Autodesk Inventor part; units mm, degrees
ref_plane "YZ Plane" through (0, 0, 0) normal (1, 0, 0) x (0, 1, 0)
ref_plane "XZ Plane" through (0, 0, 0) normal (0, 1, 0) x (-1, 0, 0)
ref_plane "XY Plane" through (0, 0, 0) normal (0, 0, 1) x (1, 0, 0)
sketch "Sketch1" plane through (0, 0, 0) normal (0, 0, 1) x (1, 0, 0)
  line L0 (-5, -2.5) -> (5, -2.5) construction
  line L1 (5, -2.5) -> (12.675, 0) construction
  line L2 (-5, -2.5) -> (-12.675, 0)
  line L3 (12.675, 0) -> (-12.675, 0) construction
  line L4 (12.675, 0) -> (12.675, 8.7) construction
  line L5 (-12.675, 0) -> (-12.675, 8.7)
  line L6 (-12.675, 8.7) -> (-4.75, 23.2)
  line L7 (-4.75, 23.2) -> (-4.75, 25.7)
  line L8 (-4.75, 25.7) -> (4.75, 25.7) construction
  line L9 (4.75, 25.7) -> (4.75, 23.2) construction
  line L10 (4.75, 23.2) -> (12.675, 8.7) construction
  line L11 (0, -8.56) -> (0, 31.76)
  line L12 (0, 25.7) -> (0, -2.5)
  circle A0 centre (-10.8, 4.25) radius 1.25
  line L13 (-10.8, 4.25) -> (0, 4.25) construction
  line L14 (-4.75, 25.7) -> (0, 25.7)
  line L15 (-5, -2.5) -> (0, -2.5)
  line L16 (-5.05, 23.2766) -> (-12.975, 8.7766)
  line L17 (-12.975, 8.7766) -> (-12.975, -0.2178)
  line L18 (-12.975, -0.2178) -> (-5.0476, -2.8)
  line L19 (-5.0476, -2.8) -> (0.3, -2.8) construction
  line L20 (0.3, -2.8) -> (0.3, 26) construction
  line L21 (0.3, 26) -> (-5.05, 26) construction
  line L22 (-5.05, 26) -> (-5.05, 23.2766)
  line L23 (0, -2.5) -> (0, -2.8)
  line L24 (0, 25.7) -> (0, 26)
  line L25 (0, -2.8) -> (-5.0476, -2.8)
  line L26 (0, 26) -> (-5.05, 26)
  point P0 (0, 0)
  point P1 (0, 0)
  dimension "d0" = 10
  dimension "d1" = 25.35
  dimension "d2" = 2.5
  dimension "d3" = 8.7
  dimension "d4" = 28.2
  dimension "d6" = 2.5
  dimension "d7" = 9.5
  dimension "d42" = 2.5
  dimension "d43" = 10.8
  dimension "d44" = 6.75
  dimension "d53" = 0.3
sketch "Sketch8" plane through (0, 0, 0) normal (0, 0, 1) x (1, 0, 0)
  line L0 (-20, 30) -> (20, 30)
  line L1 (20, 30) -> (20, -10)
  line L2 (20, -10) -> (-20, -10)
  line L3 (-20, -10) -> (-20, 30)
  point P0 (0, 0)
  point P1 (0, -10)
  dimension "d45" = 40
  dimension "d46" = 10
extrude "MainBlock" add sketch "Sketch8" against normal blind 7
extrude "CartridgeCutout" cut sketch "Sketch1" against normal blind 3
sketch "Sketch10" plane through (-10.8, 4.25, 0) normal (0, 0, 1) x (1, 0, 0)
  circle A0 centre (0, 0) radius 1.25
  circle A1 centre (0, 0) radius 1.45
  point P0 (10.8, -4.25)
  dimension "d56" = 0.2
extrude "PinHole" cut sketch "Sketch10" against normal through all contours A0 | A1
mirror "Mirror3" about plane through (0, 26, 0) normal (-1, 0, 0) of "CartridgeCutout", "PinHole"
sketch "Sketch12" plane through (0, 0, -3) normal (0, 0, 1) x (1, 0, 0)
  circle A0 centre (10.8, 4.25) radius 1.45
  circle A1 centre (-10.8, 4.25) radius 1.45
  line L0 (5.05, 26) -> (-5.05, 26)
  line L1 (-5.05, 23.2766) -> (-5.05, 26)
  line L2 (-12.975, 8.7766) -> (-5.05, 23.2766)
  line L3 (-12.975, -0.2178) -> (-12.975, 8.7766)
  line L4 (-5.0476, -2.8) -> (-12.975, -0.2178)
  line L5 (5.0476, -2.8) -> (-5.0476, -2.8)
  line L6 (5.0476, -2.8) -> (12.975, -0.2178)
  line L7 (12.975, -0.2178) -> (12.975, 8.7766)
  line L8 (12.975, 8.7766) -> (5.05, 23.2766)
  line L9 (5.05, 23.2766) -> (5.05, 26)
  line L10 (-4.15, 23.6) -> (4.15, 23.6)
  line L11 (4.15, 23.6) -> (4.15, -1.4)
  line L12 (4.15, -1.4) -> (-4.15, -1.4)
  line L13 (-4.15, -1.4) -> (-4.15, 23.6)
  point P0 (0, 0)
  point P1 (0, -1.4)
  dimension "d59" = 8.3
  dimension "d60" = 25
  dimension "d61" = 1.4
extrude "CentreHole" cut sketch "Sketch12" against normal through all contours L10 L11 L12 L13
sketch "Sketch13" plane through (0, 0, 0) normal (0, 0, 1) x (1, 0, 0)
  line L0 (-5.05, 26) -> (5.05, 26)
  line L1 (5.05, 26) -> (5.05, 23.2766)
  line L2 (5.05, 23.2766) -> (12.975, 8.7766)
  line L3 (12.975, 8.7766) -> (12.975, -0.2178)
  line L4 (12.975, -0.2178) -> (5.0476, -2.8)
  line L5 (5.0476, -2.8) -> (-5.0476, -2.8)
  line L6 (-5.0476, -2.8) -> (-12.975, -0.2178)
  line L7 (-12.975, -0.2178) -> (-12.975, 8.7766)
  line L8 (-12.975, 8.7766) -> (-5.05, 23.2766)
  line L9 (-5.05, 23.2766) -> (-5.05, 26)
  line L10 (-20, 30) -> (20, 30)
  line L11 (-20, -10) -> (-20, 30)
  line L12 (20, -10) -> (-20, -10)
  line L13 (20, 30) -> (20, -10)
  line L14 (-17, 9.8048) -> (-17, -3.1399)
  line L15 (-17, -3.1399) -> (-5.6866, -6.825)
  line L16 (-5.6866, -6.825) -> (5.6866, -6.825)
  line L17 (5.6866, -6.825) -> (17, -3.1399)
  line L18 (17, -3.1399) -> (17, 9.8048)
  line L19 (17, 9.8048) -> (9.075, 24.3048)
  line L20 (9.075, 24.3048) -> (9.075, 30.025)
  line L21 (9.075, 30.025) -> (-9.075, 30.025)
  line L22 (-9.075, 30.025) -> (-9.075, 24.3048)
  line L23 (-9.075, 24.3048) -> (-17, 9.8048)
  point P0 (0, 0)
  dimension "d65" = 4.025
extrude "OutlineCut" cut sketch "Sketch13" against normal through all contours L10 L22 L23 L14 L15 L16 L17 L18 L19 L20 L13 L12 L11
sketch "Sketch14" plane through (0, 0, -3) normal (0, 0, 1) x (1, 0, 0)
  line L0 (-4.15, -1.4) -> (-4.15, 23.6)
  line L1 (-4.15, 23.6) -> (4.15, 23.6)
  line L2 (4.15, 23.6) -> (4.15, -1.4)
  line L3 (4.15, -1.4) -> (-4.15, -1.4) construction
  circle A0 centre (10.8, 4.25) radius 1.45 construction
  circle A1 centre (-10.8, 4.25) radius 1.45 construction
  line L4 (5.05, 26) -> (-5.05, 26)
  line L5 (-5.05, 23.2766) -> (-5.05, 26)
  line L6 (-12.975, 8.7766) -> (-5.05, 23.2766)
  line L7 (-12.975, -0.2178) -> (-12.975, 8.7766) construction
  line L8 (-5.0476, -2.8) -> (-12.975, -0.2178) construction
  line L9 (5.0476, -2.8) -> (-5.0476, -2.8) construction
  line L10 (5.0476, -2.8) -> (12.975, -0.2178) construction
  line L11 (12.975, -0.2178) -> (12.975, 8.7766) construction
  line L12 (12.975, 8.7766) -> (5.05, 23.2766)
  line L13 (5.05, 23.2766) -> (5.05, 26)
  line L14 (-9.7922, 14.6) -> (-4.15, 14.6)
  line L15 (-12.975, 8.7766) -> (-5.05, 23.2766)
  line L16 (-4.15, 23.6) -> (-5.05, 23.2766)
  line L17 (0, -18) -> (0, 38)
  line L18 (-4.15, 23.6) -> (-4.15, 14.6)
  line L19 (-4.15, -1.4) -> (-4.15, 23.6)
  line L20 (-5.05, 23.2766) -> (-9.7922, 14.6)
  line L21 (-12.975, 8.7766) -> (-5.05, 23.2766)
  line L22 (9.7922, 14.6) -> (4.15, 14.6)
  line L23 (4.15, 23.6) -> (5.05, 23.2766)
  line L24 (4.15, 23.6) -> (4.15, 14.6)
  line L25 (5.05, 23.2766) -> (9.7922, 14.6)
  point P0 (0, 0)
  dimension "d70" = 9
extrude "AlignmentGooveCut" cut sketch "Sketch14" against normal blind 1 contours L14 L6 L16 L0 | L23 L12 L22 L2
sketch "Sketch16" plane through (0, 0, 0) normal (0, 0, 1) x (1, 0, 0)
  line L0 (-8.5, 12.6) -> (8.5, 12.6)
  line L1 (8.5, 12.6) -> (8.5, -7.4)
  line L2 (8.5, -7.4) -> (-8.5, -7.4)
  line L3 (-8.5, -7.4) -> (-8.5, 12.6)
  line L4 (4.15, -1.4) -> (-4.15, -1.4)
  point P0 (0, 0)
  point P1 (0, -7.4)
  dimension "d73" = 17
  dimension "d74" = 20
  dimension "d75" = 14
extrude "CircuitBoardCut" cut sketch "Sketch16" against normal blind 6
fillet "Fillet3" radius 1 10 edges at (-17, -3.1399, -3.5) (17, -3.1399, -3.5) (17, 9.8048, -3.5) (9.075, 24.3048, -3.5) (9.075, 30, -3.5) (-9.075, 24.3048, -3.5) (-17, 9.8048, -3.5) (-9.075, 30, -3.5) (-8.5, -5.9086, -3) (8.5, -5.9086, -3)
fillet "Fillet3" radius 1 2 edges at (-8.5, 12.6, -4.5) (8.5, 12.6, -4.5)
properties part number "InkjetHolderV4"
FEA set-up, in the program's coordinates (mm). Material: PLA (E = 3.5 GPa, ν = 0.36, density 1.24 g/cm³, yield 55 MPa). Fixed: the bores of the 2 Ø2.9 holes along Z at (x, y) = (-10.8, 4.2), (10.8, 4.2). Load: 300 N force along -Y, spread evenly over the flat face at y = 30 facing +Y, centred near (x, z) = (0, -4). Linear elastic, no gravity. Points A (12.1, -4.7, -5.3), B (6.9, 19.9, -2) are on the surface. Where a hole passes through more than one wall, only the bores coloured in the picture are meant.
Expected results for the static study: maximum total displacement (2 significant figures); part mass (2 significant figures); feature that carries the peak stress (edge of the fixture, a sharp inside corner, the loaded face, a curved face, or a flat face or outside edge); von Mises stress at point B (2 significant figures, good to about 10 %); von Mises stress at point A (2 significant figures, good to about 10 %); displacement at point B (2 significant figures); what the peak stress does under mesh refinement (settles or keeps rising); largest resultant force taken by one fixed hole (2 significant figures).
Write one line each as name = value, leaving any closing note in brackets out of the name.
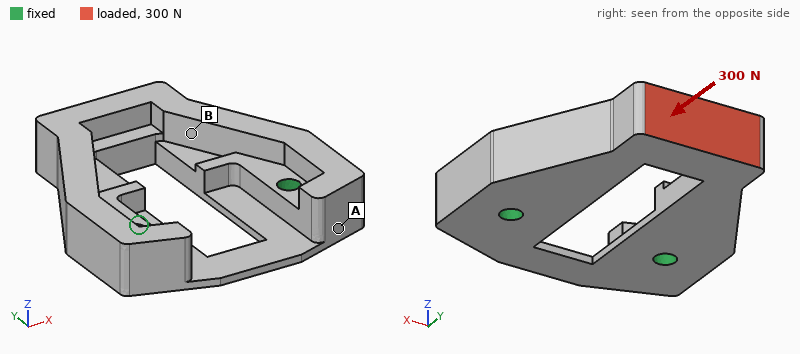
maximum total displacement = 0.19 mm
part mass = 4.4 g
feature that carries the peak stress = edge of the fixture
von Mises stress at point B = 5.6 MPa
von Mises stress at point A = 2.0 MPa
displacement at point B = 0.087 mm
what the peak stress does under mesh refinement = keeps rising
largest resultant force taken by one fixed hole = 160 N
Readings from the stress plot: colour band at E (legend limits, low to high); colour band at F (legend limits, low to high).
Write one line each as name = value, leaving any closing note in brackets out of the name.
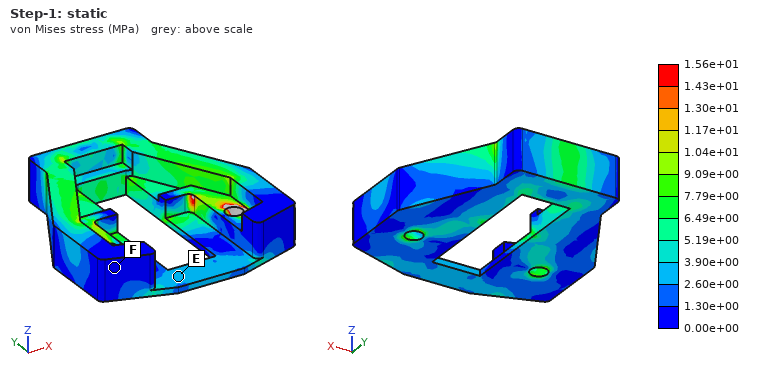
colour band at E = 2.60e+00 to 3.90e+00 MPa
colour band at F = 0.00e+00 to 1.30e+00 MPa
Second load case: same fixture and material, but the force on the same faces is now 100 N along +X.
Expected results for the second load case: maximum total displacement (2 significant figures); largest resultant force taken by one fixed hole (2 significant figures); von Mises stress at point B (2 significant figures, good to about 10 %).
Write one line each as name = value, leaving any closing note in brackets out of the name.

maximum total displacement = 0.12 mm
largest resultant force taken by one fixed hole = 92 N
von Mises stress at point B = 4.5 MPa
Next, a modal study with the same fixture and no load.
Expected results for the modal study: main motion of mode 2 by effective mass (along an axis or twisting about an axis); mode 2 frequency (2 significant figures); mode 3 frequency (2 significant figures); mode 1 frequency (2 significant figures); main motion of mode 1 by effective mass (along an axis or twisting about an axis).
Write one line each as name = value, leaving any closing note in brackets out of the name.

main motion of mode 2 by effective mass = along X
mode 2 frequency = 3700 Hz
mode 3 frequency = 4800 Hz
mode 1 frequency = 1800 Hz
main motion of mode 1 by effective mass = along Z
